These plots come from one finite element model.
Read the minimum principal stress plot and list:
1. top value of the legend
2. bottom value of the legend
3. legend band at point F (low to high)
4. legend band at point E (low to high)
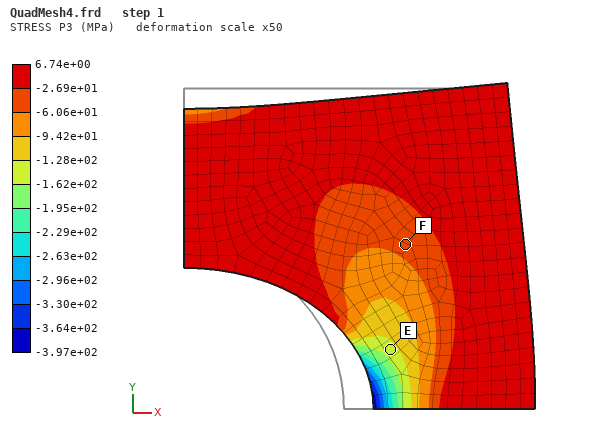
6.74e+00 MPa
-3.97e+02 MPa
-6.06e+01 to -2.69e+01 MPa
-1.62e+02 to -1.28e+02 MPa
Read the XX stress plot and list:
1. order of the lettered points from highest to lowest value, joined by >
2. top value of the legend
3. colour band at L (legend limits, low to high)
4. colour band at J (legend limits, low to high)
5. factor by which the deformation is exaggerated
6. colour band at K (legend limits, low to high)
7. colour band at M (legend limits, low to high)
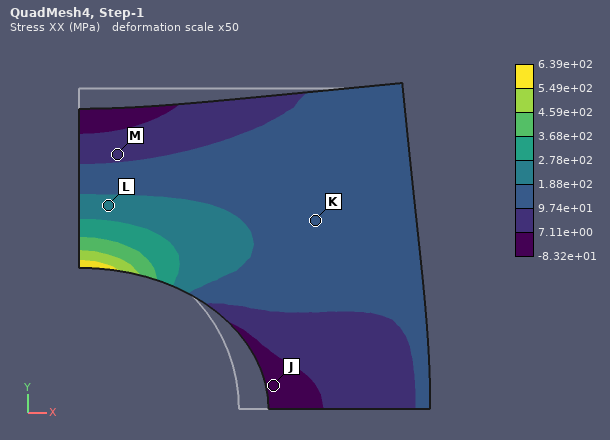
L > K > M > J
6.39e+02 MPa
1.88e+02 to 2.78e+02 MPa
-8.32e+01 to 7.11e+00 MPa
50
9.74e+01 to 1.88e+02 MPa
7.11e+00 to 9.74e+01 MPa
